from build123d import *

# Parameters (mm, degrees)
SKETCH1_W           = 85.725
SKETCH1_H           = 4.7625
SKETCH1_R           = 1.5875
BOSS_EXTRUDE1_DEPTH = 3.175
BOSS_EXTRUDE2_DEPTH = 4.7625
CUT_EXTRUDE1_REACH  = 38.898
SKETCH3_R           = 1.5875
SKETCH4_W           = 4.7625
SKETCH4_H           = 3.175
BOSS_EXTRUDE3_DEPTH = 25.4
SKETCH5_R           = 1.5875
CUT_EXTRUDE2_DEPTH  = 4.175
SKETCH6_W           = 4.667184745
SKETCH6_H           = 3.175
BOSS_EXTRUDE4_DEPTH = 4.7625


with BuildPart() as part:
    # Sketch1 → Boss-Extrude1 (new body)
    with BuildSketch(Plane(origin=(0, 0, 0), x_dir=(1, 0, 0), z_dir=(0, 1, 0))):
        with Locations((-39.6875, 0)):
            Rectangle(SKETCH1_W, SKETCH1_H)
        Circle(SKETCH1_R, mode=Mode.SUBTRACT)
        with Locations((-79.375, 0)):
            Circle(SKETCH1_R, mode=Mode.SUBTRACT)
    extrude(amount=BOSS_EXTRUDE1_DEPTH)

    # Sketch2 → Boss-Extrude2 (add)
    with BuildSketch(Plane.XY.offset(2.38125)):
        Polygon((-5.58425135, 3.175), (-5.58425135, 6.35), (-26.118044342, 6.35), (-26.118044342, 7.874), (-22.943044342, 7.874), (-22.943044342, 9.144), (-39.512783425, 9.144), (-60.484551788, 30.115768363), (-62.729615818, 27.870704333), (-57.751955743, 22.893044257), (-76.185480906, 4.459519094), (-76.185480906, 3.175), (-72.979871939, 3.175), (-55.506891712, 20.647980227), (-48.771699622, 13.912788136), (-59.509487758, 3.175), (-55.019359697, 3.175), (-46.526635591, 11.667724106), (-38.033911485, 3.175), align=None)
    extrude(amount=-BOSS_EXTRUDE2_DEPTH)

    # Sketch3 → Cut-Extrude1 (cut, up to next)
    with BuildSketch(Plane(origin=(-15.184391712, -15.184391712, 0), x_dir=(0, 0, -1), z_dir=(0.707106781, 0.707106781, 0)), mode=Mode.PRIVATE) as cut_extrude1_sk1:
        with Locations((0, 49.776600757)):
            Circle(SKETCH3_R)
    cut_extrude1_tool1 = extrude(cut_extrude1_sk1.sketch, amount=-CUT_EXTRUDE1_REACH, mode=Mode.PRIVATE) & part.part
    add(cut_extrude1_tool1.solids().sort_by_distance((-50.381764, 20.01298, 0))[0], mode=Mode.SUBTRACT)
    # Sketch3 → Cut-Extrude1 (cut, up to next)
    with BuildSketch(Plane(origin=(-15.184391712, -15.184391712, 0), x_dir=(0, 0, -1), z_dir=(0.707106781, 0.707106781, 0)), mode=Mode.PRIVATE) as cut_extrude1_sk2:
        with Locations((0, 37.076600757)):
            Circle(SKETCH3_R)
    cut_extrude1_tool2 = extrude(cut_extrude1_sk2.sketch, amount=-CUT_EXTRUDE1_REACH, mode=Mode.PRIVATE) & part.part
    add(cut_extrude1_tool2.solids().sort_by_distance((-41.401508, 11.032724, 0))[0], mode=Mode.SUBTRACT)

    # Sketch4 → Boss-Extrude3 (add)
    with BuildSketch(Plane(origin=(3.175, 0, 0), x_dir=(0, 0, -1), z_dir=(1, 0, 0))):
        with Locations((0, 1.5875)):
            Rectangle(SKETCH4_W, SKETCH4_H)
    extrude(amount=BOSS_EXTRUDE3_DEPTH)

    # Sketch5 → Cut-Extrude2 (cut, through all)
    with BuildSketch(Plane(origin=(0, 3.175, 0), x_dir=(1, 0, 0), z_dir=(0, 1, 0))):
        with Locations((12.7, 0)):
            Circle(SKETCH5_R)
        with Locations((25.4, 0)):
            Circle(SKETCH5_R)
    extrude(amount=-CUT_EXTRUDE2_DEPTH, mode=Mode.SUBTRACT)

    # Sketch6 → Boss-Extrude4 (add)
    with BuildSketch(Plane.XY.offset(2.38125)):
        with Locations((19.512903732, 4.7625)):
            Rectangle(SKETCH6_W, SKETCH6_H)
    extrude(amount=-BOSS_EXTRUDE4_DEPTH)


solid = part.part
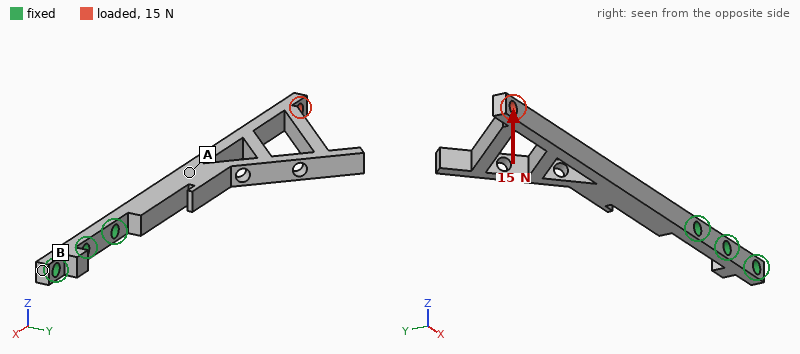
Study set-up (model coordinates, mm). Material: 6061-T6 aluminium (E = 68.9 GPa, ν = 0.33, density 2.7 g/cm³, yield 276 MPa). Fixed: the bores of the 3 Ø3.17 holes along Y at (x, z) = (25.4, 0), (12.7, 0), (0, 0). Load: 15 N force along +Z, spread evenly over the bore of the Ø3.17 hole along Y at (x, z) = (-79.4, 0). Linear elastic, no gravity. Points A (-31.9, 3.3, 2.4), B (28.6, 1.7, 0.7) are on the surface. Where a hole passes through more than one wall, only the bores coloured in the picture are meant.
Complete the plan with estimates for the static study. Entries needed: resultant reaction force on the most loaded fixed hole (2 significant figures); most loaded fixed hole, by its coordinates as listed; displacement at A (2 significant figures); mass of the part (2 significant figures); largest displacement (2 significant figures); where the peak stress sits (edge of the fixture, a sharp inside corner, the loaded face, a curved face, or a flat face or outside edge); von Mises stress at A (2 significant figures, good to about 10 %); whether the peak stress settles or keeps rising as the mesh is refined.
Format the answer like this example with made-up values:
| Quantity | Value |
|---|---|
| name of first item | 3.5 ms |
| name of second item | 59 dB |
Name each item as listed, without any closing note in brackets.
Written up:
| Quantity | Value |
|---|---|
| resultant reaction force on the most loaded fixed hole | 19 N |
| most loaded fixed hole, by its coordinates as listed | (0, 0) |
| displacement at A | 0.19 mm |
| mass of the part | 9.1 g |
| largest displacement | 0.84 mm |
| where the peak stress sits | edge of the fixture |
| von Mises stress at A | 23 MPa |
| whether the peak stress settles or keeps rising as the mesh is refined | keeps rising |
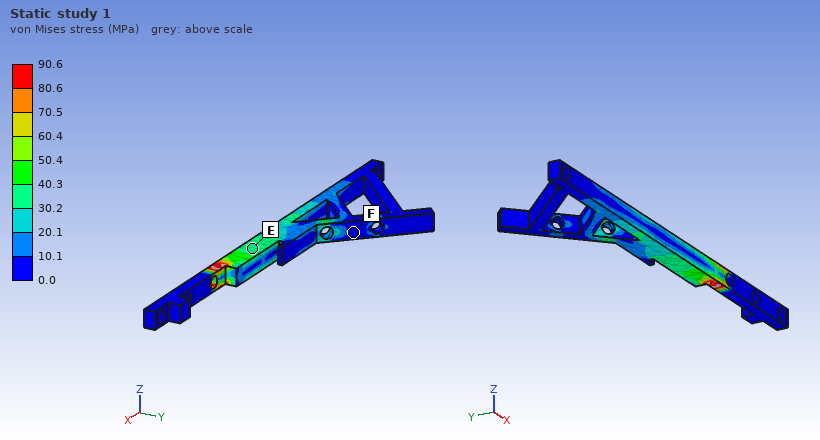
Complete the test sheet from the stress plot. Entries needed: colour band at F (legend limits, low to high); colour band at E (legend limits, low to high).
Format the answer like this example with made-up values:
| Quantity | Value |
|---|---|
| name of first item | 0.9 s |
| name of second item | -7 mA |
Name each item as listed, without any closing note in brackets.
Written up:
| Quantity | Value |
|---|---|
| colour band at F | 0.0 to 10.1 MPa |
| colour band at E | 30.2 to 40.3 MPa |
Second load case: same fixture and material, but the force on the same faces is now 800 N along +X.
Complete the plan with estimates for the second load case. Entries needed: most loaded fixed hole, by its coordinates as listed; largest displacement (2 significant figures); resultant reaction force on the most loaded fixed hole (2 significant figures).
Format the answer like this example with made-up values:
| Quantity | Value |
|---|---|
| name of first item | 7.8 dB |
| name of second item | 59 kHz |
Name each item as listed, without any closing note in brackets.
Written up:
| Quantity | Value |
|---|---|
| most loaded fixed hole, by its coordinates as listed | (0, 0) |
| largest displacement | 0.39 mm |
| resultant reaction force on the most loaded fixed hole | 800 N |
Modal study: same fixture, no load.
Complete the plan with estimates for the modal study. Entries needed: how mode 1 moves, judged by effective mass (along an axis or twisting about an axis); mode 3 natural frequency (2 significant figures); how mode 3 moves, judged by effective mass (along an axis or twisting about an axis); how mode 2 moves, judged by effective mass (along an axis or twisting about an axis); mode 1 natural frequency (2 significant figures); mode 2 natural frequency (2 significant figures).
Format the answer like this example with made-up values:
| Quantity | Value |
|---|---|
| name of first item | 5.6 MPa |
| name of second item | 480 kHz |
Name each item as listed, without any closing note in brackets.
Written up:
| Quantity | Value |
|---|---|
| how mode 1 moves, judged by effective mass | along Y |
| mode 3 natural frequency | 1900 Hz |
| how mode 3 moves, judged by effective mass | twisting about X |
| how mode 2 moves, judged by effective mass | along Z |
| mode 1 natural frequency | 430 Hz |
| mode 2 natural frequency | 480 Hz |
